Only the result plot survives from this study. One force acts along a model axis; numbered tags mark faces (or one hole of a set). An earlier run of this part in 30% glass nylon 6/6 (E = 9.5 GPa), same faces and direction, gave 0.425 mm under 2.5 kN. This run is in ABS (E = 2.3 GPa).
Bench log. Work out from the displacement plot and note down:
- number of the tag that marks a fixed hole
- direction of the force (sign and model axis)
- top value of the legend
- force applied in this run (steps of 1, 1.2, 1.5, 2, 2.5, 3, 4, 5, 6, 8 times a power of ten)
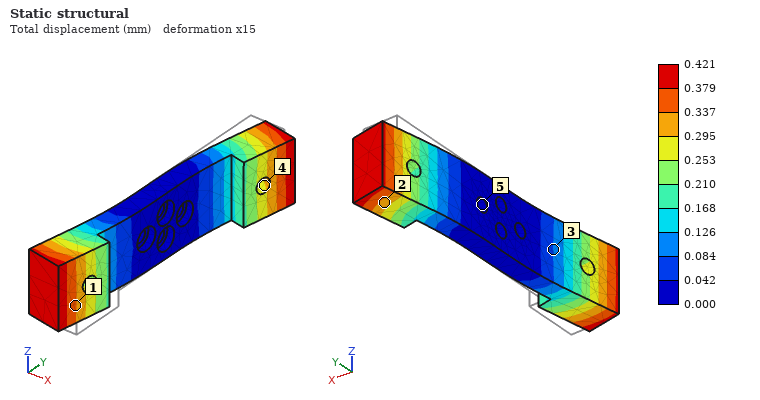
5
-Y
0.421 mm
600 N
